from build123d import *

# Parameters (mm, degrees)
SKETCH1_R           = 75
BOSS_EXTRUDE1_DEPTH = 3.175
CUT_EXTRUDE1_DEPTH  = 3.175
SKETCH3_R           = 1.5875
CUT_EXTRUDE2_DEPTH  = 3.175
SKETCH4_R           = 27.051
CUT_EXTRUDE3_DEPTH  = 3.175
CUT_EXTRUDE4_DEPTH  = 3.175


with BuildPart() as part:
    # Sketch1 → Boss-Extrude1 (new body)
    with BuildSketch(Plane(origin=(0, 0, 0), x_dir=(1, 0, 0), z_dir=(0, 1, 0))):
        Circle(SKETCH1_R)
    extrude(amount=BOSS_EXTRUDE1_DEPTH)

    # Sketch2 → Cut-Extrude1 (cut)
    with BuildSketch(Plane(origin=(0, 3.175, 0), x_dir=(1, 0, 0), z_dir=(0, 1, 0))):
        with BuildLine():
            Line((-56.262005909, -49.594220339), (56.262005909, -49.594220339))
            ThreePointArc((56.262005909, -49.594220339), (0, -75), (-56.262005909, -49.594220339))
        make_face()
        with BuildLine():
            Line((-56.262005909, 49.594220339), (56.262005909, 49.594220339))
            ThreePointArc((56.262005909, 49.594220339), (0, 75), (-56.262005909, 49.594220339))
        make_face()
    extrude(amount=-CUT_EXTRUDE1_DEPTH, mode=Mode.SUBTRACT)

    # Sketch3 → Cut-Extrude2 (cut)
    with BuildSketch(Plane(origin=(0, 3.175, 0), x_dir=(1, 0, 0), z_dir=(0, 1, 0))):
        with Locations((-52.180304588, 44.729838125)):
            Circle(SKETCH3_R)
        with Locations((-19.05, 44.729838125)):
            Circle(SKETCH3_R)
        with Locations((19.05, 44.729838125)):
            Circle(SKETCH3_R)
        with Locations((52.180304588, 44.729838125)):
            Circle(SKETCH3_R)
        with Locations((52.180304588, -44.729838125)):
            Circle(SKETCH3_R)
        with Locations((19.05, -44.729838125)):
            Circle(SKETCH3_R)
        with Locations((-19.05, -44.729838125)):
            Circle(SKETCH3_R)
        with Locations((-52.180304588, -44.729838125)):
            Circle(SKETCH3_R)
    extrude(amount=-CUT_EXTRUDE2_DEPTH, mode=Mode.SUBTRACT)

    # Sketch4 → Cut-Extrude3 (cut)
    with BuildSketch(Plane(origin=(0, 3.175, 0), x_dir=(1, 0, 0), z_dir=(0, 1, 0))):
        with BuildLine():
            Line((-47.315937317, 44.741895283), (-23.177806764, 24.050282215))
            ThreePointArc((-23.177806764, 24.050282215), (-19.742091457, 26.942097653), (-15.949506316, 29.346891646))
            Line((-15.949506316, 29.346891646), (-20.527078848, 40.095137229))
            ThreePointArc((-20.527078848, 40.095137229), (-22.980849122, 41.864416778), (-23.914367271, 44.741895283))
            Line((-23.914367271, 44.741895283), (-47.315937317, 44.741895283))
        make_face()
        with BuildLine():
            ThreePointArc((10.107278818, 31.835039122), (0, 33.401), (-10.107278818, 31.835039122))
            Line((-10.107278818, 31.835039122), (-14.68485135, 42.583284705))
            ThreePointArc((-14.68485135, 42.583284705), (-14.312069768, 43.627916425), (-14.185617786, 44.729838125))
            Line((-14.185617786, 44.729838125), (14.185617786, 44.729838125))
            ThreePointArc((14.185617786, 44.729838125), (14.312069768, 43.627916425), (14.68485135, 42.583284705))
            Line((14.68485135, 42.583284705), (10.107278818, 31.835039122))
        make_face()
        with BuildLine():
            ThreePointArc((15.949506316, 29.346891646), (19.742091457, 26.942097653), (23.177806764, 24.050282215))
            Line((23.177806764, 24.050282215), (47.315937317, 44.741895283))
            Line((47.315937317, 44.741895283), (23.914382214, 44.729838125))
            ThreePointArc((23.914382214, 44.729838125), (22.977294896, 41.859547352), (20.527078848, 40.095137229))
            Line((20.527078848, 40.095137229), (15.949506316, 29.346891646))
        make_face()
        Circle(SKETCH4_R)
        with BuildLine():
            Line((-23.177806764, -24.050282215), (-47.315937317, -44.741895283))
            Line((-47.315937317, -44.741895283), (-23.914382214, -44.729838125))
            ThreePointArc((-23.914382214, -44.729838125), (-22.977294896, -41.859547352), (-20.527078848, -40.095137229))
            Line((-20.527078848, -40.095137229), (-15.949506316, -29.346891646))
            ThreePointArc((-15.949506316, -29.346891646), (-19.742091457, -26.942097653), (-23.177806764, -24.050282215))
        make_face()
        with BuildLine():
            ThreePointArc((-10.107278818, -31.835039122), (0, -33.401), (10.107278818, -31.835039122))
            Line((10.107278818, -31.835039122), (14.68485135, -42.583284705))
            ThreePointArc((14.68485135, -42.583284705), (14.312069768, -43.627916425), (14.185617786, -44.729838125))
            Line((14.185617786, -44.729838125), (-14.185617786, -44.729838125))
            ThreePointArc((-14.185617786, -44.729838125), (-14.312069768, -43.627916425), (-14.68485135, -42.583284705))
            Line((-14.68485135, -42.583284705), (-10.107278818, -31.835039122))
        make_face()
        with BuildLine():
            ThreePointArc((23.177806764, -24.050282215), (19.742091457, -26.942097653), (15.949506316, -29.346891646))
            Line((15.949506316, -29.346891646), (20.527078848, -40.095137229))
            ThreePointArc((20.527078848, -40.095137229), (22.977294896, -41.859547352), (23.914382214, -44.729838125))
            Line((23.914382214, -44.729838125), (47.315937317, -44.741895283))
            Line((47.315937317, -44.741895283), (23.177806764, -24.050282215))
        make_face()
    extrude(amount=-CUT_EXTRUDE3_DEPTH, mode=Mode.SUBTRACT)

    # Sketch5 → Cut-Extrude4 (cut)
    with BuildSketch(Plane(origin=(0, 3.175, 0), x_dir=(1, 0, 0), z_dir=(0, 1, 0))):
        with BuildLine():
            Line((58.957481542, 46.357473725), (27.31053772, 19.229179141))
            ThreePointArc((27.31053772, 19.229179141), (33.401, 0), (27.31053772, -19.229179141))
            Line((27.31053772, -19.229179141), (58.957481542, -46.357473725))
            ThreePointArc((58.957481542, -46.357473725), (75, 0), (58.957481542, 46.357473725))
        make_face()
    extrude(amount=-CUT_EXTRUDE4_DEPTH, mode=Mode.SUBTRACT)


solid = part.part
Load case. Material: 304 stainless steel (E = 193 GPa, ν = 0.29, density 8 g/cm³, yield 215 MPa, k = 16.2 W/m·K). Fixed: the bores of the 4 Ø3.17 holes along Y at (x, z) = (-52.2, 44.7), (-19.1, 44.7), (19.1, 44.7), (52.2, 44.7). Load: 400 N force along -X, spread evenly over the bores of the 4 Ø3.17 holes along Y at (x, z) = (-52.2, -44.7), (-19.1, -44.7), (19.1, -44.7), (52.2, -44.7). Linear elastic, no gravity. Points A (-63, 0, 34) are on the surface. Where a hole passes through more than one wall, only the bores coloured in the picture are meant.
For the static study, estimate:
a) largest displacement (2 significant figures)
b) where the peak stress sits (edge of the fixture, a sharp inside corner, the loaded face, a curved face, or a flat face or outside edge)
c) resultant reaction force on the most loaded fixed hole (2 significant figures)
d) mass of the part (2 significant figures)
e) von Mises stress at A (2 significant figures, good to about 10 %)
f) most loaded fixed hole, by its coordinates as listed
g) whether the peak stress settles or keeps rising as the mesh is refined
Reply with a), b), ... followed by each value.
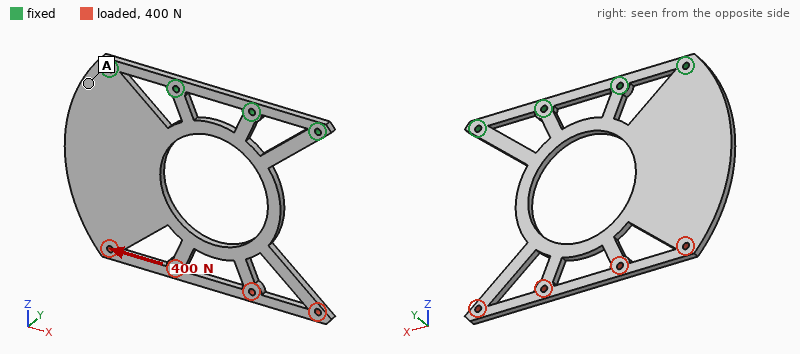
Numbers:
a) 36 µm
b) edge of the fixture
c) 580 N
d) 170 g
e) 9.3 MPa
f) (-52.2, 44.7)
g) keeps rising
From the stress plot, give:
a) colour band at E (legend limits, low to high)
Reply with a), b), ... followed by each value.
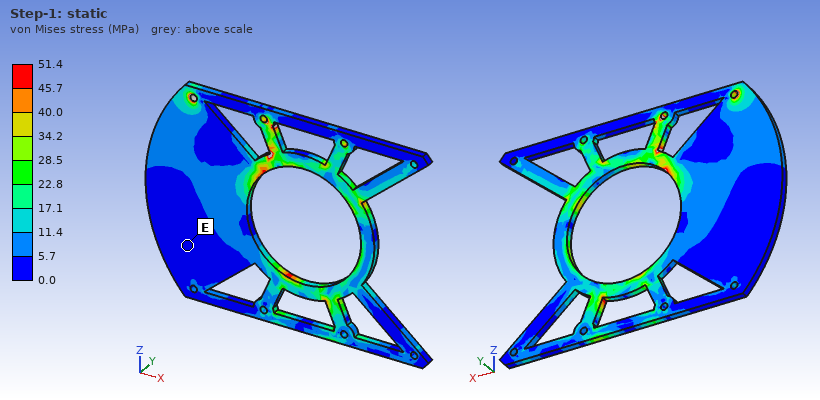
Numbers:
a) 0.0 to 5.7 MPa
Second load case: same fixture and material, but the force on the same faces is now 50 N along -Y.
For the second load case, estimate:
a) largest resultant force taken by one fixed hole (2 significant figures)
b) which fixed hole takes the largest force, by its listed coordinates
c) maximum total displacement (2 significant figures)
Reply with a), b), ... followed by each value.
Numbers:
a) 20 N
b) (-19.1, 44.7)
c) 0.90 mm
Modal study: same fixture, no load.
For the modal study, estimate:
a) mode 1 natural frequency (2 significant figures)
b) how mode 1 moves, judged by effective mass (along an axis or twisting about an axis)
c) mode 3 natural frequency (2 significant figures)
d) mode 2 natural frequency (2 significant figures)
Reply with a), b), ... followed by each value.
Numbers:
a) 220 Hz
b) along Y
c) 1100 Hz
d) 410 Hz
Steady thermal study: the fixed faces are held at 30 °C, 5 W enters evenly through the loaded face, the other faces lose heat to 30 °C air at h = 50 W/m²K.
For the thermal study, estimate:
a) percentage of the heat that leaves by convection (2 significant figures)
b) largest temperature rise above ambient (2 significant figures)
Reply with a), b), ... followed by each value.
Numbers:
a) 99 %
b) 43 K
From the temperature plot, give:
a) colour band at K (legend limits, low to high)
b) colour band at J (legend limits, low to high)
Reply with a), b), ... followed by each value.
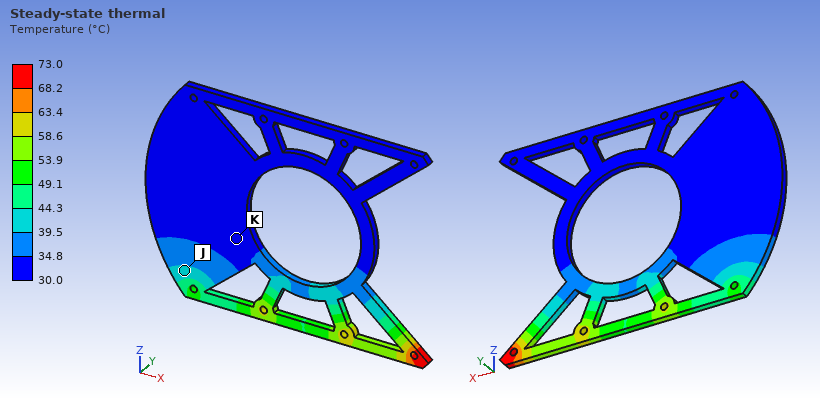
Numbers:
a) 30.0 to 34.8 °C
b) 39.5 to 44.3 °C
